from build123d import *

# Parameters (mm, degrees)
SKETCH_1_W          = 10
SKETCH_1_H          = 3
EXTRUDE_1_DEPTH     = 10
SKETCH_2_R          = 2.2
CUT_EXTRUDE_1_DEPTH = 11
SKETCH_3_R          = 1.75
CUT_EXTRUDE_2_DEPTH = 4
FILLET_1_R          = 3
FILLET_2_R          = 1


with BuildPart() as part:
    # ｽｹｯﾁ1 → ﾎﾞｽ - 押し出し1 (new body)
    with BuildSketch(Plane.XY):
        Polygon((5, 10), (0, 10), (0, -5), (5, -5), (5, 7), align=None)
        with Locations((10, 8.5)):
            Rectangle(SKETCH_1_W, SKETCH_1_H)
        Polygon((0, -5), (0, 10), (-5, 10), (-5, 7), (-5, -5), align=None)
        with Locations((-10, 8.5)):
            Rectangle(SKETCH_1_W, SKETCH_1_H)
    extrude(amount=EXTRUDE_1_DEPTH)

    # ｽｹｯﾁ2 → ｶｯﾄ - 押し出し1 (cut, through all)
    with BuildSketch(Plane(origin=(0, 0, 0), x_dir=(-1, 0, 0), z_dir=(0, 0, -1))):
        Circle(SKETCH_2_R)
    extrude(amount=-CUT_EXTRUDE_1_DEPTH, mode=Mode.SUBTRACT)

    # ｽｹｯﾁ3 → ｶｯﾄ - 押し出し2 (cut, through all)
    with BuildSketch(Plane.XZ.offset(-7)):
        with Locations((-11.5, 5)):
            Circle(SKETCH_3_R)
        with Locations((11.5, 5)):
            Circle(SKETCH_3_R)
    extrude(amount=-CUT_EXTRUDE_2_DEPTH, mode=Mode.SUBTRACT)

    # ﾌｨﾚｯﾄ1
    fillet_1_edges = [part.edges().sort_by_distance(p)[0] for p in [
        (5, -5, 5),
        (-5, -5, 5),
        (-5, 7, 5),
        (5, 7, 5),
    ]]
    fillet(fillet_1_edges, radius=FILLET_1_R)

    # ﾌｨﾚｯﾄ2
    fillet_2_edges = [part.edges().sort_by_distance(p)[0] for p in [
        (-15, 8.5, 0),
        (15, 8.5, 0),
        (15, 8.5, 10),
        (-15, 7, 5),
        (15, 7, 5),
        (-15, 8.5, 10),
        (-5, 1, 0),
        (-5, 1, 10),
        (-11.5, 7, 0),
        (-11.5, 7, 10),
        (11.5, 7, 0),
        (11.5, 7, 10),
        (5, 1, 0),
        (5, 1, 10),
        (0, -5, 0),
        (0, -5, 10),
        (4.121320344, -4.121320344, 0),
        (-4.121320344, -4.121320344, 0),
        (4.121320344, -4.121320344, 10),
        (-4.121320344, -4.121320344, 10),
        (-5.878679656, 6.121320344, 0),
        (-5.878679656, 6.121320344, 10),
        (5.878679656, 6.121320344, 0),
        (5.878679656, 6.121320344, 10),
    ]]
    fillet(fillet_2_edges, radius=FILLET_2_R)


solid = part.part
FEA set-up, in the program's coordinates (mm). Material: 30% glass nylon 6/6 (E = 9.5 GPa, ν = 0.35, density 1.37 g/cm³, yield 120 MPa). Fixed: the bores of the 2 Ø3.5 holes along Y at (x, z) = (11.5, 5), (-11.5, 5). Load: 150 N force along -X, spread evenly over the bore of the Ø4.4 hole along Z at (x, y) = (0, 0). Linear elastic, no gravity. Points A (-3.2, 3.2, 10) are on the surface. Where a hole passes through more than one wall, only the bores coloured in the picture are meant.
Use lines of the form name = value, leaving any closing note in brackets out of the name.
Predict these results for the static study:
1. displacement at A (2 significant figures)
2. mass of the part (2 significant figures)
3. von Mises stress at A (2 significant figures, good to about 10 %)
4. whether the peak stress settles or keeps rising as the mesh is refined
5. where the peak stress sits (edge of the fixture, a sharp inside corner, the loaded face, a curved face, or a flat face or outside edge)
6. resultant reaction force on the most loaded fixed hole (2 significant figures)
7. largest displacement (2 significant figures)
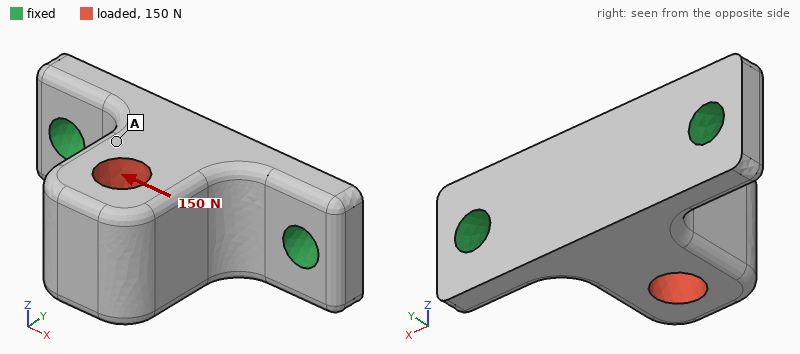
displacement at A = 9.6 µm
mass of the part = 2.6 g
von Mises stress at A = 2.3 MPa
whether the peak stress settles or keeps rising as the mesh is refined = keeps rising
where the peak stress sits = edge of the fixture
resultant reaction force on the most loaded fixed hole = 110 N
largest displacement = 26 µm
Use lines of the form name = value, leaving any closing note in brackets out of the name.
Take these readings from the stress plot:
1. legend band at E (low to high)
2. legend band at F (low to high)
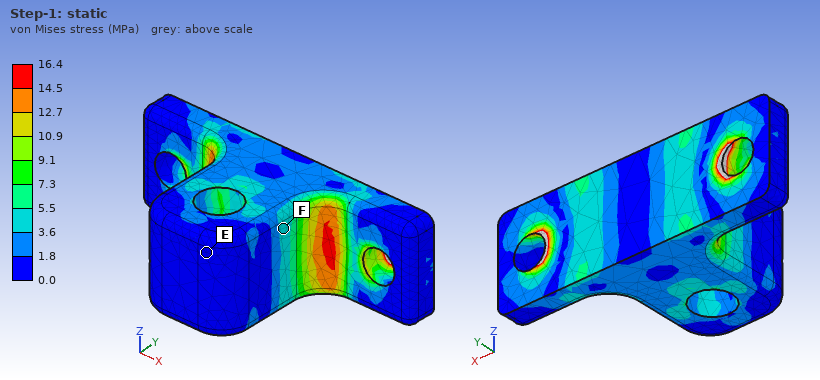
legend band at E = 0.0 to 1.8 MPa
legend band at F = 3.6 to 5.5 MPa
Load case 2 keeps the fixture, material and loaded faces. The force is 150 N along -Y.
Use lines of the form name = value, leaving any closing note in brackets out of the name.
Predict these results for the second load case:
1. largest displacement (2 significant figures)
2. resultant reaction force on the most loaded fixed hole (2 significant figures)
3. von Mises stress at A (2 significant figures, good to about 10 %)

largest displacement = 13 µm
resultant reaction force on the most loaded fixed hole = 86 N
von Mises stress at A = 2.3 MPa
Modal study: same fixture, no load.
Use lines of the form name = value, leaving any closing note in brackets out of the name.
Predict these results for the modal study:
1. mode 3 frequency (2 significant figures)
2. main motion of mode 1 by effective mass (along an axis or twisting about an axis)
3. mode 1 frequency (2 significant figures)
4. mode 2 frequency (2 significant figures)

mode 3 frequency = 13 kHz
main motion of mode 1 by effective mass = along Z
mode 1 frequency = 5400 Hz
mode 2 frequency = 13 kHz
